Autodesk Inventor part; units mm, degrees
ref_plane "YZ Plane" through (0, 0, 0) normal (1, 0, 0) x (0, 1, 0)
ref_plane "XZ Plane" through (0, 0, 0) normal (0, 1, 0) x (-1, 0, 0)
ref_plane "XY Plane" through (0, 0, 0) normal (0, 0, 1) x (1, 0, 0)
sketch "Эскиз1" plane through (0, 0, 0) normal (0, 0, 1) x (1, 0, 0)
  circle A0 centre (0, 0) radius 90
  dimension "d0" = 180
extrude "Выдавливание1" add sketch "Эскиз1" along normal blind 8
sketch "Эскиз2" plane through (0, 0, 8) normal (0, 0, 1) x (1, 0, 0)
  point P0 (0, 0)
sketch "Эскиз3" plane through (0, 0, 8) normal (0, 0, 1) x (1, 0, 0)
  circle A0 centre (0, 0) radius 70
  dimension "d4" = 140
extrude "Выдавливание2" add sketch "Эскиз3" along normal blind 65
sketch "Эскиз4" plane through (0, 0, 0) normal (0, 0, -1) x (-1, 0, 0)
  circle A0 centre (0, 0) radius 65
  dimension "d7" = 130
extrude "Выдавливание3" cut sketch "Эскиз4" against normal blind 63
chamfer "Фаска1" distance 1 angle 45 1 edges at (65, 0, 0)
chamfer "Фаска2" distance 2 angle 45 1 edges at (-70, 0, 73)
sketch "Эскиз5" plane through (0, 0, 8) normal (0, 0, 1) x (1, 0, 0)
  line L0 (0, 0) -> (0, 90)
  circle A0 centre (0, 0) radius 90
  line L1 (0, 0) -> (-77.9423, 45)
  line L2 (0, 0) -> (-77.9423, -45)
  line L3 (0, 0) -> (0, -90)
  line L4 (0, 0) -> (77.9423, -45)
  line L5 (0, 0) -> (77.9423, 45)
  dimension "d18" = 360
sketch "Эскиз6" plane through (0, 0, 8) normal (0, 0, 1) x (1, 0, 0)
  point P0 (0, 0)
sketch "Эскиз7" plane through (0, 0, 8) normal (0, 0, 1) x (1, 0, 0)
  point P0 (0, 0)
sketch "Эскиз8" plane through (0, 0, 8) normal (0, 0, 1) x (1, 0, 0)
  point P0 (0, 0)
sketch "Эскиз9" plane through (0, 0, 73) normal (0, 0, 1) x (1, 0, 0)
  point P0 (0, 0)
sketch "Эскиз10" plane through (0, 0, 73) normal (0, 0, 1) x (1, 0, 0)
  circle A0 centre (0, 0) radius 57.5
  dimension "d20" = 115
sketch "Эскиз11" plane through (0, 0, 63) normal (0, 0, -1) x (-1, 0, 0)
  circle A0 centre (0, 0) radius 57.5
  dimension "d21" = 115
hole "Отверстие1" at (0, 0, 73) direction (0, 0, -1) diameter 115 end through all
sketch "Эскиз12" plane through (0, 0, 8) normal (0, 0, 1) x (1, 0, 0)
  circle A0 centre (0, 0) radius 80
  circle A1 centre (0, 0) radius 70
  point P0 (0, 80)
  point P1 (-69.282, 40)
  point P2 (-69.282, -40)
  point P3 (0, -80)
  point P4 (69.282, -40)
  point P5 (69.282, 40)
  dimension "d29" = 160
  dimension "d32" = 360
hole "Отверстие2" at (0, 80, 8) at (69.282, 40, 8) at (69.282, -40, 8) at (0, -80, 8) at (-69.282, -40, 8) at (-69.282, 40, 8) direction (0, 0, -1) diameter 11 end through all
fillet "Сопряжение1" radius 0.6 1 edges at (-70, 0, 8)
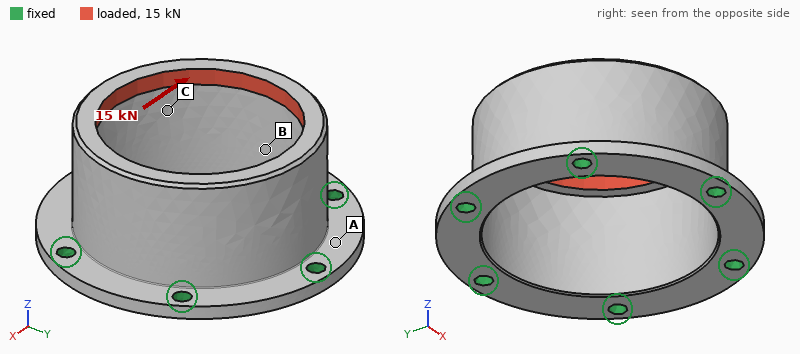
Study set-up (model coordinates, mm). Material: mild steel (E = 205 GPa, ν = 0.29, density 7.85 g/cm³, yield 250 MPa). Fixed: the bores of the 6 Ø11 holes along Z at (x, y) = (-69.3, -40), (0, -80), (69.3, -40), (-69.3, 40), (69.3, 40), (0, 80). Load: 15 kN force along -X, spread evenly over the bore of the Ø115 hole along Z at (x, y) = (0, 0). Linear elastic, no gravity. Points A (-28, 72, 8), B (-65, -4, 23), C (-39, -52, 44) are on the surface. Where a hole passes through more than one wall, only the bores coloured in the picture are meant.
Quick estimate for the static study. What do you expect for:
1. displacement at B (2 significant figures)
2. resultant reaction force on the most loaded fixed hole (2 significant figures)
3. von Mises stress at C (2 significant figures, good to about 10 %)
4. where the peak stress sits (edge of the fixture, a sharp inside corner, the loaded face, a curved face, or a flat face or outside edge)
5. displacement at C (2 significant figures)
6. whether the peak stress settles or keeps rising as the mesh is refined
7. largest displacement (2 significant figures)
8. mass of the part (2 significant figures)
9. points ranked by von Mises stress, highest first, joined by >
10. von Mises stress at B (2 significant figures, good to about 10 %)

8.3 µm
4.4 kN
26 MPa
edge of the fixture
12 µm
keeps rising
28 µm
2.0 kg
C > B > A
13 MPa
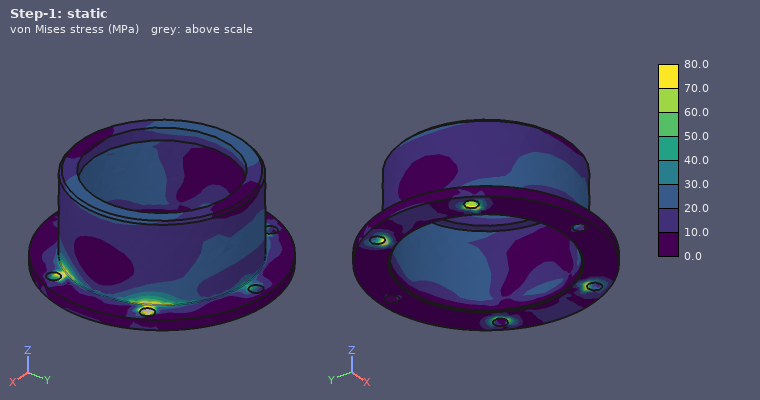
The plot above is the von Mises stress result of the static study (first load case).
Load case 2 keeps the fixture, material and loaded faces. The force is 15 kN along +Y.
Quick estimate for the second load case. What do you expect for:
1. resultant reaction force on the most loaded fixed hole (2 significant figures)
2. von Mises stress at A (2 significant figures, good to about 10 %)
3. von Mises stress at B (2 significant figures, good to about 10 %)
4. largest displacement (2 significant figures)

4.7 kN
13 MPa
26 MPa
28 µm
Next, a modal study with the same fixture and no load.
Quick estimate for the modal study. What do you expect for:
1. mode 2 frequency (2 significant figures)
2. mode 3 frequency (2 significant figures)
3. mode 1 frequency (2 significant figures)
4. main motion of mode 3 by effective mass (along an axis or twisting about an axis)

3000 Hz
4800 Hz
3000 Hz
along Y
